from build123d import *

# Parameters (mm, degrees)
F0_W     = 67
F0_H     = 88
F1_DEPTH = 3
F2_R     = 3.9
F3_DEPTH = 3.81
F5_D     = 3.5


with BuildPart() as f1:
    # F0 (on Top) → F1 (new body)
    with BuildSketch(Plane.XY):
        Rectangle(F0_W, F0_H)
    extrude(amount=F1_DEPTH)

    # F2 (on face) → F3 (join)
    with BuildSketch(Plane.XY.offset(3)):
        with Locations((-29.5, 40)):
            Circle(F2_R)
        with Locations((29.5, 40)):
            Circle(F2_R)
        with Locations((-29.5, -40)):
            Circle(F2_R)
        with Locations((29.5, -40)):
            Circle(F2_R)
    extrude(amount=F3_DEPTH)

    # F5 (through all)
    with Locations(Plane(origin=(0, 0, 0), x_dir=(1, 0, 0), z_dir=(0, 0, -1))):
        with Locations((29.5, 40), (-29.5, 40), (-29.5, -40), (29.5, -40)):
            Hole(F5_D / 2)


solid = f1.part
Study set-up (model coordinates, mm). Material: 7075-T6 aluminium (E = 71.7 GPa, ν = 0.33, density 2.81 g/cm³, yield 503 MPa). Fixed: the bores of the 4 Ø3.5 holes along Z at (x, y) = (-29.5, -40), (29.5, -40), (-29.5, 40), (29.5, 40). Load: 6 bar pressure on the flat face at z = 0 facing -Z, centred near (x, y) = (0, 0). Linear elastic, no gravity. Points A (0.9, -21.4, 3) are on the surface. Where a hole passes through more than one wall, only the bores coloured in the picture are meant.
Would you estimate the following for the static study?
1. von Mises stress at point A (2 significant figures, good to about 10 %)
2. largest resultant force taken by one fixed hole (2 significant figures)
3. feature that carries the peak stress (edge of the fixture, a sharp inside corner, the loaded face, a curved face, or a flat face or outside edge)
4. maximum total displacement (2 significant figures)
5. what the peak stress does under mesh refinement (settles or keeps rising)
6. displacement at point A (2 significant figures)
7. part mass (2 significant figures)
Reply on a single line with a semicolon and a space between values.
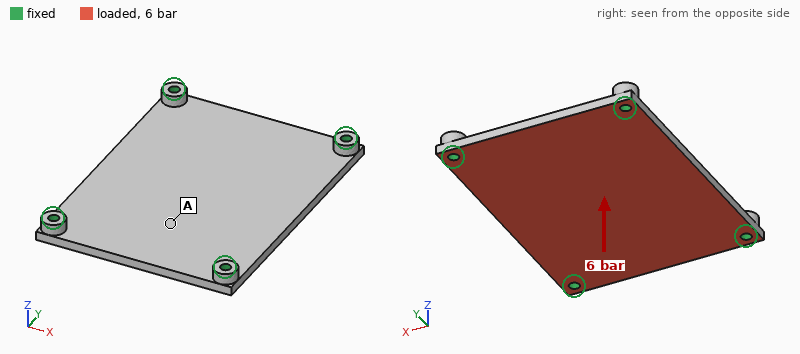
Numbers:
74 MPa; 920 N; edge of the fixture; 0.62 mm; keeps rising; 0.44 mm; 51 g
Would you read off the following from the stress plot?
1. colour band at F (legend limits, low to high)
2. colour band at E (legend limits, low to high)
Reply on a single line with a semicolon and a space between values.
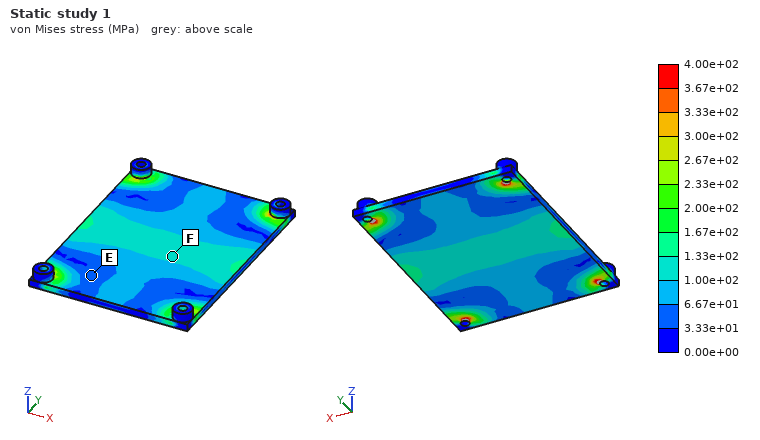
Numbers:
1.00e+02 to 1.33e+02 MPa; 3.33e+01 to 6.67e+01 MPa
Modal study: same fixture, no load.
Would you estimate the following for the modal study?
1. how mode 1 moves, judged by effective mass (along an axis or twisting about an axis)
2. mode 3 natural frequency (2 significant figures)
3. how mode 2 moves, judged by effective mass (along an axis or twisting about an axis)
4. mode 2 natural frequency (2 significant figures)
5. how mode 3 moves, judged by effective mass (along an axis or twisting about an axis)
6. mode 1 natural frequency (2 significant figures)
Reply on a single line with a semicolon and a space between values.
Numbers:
along Z; 4500 Hz; twisting about Y; 3200 Hz; twisting about X; 2000 Hz
